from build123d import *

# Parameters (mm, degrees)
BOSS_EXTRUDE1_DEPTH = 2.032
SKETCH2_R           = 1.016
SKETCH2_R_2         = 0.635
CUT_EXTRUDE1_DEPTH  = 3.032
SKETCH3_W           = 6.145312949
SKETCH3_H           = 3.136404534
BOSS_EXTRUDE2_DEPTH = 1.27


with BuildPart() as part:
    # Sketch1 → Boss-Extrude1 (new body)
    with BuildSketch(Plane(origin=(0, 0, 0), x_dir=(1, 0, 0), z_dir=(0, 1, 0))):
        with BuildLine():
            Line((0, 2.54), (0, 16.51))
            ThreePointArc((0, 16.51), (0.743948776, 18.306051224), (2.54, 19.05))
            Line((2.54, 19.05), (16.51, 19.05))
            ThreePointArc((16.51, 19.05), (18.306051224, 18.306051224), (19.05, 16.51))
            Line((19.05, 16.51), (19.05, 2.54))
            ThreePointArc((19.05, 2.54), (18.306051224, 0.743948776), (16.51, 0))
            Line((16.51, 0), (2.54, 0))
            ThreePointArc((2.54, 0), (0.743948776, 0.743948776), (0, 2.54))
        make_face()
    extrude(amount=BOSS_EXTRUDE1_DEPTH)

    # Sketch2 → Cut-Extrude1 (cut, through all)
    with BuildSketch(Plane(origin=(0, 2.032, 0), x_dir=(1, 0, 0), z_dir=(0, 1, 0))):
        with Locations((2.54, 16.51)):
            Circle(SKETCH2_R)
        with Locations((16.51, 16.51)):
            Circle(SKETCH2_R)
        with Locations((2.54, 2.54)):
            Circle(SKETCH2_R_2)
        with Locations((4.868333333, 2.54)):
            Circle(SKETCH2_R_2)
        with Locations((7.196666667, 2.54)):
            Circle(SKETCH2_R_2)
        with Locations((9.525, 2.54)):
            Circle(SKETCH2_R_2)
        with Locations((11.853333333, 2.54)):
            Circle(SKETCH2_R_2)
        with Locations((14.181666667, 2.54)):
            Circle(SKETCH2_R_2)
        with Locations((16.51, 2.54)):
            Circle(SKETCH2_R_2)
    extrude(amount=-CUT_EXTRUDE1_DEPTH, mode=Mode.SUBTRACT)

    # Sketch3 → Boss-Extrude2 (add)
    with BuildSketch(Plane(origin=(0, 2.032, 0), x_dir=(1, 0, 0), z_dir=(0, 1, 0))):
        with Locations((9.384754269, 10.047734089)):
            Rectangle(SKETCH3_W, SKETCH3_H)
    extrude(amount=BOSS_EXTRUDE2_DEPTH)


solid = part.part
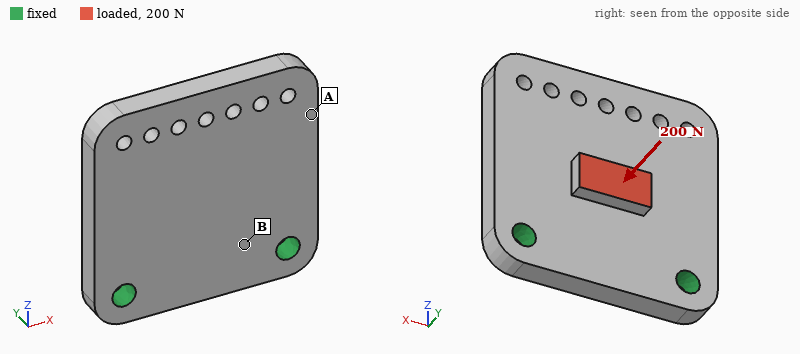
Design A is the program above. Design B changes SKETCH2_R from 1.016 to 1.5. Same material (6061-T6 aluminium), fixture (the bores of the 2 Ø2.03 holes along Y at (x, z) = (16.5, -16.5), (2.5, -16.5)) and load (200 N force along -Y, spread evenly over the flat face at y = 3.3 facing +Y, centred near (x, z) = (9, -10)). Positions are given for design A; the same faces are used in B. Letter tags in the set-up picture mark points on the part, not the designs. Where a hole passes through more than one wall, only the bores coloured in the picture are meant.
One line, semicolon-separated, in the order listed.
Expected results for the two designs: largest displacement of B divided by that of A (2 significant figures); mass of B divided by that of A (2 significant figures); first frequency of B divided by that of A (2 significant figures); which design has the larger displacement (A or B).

0.79; 0.98; 1.1; A
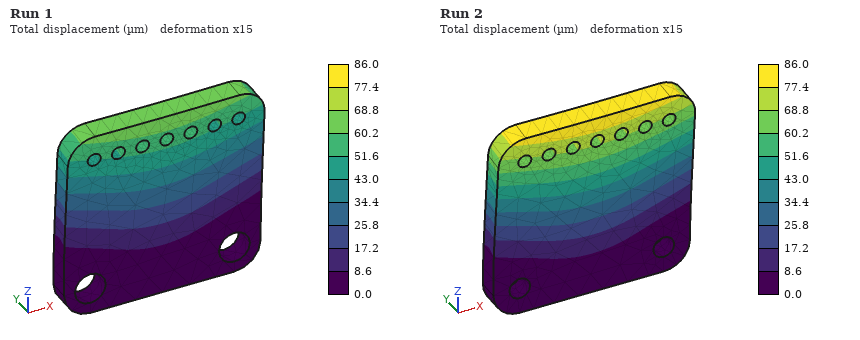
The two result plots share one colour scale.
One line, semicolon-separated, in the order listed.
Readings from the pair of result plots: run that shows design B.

Run 1
